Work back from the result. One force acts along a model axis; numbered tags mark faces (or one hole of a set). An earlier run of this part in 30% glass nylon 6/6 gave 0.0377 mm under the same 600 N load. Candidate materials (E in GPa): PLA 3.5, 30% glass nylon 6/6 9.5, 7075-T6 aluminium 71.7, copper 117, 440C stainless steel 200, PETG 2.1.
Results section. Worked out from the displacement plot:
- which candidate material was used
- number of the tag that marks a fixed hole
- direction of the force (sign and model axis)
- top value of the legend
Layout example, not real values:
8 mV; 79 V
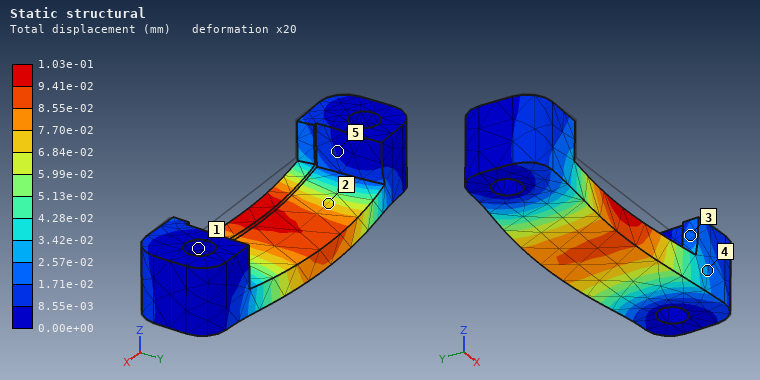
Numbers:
PLA; 1; +Y; 1.03e-01 mm
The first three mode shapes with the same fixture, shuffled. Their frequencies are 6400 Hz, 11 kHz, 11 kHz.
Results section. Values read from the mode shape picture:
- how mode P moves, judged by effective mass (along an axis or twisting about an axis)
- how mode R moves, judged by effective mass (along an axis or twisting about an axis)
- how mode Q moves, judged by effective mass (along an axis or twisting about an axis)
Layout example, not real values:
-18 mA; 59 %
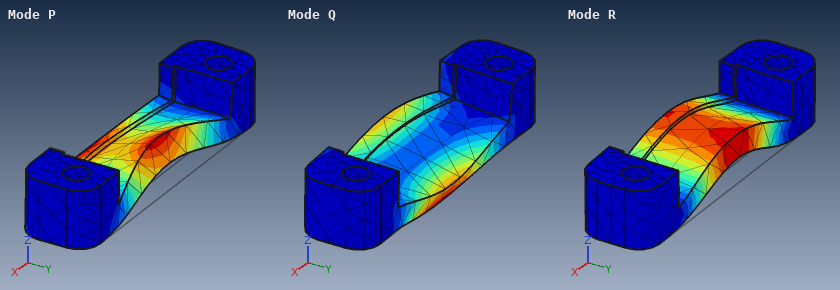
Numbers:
along Y; along Z; along Y
